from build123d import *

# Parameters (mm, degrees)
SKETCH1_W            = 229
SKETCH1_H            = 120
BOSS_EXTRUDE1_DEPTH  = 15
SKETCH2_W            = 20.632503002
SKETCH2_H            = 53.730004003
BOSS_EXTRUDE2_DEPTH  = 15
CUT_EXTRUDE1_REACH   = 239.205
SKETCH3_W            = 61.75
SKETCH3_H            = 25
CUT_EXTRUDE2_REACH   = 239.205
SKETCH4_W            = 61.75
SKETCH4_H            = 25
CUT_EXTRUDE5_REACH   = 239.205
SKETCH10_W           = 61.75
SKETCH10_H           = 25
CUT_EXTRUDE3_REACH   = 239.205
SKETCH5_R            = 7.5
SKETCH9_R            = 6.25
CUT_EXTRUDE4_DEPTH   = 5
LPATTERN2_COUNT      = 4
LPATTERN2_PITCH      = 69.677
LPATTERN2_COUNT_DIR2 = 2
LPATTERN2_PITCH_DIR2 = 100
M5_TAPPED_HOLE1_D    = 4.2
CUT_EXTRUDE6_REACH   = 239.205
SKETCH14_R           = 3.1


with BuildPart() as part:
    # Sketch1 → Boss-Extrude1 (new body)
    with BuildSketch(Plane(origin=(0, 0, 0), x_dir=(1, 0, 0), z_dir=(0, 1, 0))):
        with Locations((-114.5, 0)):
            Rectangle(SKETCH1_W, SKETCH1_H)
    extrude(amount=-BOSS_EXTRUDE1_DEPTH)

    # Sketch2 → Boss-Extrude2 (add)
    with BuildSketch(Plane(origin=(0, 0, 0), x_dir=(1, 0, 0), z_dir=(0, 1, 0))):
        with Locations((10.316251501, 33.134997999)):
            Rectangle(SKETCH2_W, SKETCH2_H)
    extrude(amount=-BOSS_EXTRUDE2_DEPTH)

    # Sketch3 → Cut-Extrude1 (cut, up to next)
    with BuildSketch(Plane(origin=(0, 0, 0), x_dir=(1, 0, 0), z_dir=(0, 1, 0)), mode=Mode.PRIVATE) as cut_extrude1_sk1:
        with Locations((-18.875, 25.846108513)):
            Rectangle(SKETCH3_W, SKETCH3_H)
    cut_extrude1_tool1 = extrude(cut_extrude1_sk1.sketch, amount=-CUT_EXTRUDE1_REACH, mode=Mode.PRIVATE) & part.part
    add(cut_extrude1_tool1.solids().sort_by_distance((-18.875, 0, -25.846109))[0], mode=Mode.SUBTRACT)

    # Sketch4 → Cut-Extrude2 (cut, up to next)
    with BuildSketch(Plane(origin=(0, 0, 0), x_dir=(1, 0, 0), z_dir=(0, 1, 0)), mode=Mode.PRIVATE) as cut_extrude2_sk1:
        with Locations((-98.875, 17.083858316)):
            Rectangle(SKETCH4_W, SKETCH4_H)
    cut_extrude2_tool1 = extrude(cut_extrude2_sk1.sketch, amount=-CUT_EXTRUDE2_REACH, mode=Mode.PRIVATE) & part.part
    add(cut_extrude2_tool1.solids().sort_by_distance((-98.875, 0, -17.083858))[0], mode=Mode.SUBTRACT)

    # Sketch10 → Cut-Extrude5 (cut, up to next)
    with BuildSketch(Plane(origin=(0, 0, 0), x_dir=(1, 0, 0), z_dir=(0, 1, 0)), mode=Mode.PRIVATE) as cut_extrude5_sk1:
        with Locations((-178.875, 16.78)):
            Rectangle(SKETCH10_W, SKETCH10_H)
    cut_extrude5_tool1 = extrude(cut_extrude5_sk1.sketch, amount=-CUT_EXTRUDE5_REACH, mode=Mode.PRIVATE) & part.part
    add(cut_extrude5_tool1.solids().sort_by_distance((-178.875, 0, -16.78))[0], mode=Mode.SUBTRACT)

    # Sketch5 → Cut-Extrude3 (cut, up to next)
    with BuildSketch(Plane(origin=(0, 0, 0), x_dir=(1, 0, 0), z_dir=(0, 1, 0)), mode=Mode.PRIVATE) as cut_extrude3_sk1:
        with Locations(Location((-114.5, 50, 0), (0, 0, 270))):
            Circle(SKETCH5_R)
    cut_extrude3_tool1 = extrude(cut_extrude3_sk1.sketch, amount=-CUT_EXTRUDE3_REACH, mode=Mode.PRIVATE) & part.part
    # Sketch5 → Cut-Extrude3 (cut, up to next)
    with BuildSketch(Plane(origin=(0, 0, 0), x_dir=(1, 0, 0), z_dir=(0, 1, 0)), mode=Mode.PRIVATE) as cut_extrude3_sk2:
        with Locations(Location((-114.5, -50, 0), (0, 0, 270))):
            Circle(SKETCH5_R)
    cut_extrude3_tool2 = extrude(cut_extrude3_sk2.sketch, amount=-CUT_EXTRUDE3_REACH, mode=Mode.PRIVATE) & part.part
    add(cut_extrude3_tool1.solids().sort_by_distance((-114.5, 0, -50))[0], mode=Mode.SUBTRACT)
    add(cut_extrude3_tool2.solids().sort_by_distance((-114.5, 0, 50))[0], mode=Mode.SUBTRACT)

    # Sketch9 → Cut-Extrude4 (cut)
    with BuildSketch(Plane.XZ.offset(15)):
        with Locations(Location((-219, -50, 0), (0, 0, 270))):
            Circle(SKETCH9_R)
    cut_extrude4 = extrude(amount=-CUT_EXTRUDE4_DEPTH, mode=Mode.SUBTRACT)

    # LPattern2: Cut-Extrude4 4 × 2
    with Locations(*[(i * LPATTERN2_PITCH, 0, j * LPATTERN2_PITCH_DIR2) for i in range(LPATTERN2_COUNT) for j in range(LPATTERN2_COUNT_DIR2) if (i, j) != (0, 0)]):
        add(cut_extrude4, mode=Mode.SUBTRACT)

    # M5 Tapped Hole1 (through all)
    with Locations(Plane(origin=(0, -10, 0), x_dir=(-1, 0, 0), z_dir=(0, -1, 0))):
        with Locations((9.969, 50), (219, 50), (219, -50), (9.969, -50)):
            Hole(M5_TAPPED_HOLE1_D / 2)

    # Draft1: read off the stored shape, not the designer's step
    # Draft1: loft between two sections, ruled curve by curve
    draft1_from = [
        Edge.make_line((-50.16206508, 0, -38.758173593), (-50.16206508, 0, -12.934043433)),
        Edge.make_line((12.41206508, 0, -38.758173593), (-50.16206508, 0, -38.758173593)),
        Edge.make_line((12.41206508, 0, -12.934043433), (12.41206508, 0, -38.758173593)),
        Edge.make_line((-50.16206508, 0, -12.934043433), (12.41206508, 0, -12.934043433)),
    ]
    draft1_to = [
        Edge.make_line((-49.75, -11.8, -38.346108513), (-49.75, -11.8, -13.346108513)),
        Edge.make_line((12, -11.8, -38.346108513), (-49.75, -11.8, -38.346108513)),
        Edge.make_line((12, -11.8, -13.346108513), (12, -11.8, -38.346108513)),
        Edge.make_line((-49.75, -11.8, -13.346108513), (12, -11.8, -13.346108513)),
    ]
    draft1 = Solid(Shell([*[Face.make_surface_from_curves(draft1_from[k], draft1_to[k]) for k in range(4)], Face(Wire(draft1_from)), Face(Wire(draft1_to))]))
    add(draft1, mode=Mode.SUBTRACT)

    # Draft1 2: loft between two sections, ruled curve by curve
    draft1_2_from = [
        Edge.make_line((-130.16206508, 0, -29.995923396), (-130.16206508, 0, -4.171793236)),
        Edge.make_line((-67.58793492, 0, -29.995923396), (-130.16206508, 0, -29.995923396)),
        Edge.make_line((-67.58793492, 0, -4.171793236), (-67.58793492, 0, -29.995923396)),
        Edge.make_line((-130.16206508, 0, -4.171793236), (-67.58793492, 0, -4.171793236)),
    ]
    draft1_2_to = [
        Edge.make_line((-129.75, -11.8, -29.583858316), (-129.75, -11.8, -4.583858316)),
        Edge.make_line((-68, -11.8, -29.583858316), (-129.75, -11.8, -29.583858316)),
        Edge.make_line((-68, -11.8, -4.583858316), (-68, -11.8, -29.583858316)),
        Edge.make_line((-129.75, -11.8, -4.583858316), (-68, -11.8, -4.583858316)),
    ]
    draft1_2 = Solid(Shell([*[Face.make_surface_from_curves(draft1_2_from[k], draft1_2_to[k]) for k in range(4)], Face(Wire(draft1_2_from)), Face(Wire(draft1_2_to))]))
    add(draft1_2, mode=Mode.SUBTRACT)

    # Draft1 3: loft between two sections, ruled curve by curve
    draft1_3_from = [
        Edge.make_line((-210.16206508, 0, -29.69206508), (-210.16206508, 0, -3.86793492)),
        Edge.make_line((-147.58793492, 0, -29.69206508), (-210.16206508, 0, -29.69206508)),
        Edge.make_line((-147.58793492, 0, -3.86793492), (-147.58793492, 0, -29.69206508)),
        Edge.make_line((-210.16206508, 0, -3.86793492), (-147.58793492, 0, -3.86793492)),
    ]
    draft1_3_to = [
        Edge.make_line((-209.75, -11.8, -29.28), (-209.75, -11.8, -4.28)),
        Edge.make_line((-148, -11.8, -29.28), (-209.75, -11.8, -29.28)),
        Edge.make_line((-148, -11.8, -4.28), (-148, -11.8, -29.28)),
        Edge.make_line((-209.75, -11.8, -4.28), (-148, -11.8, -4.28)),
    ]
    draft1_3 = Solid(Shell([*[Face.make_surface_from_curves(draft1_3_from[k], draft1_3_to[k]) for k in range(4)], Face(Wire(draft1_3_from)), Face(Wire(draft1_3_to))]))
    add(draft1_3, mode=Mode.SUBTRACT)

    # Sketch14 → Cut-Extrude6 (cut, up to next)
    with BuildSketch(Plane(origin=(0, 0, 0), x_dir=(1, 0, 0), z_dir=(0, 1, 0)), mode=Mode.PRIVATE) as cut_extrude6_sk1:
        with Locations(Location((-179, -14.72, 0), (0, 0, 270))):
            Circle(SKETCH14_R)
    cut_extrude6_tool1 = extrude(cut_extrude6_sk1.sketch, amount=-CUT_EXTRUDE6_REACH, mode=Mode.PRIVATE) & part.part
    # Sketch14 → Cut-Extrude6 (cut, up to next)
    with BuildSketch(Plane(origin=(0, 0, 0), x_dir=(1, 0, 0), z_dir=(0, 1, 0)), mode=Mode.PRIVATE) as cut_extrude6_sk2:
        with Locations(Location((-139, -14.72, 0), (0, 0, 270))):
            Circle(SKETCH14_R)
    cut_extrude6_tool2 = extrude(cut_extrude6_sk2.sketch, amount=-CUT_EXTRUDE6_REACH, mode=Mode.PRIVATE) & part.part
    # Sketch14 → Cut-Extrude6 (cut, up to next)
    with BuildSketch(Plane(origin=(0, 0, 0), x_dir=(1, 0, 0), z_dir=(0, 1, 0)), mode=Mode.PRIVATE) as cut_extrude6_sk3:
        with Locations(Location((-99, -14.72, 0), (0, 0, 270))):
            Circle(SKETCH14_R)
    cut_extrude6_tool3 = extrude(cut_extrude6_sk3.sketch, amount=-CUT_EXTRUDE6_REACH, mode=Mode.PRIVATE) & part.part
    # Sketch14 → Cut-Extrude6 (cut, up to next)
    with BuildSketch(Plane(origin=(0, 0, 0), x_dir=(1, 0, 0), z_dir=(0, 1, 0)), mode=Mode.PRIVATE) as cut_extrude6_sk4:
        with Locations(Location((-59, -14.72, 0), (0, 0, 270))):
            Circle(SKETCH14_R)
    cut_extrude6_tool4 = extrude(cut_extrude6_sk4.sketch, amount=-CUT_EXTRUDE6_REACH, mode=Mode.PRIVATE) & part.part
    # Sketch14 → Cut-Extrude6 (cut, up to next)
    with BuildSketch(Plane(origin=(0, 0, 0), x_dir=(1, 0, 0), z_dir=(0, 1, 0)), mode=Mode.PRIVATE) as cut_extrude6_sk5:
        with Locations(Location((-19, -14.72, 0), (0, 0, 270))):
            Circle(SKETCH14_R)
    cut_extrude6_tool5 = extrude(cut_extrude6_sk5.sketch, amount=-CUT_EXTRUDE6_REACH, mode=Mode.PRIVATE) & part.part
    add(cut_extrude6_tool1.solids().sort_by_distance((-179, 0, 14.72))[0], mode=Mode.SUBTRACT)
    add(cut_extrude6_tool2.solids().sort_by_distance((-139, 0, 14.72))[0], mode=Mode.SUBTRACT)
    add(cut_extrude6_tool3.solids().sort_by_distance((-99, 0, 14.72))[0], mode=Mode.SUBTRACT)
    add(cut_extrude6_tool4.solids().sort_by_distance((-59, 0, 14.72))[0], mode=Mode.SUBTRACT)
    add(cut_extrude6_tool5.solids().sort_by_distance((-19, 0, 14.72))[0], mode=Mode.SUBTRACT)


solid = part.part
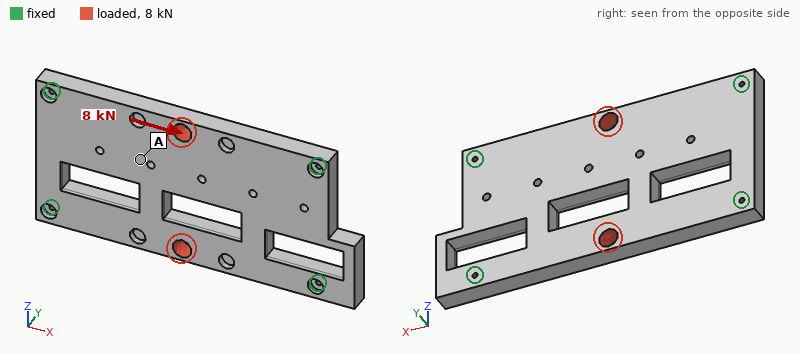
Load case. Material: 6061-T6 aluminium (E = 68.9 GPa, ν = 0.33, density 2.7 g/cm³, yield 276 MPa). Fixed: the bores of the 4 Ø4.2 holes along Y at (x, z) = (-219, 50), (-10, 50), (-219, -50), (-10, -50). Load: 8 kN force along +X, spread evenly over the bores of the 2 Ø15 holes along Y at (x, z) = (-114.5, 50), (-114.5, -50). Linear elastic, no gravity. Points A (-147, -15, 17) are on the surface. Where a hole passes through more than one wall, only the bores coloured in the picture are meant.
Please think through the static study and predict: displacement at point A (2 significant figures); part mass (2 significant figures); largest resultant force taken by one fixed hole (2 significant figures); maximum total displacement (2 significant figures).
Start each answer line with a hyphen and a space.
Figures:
- 5.3 µm
- 930 g
- 2.1 kN
- 10 µm
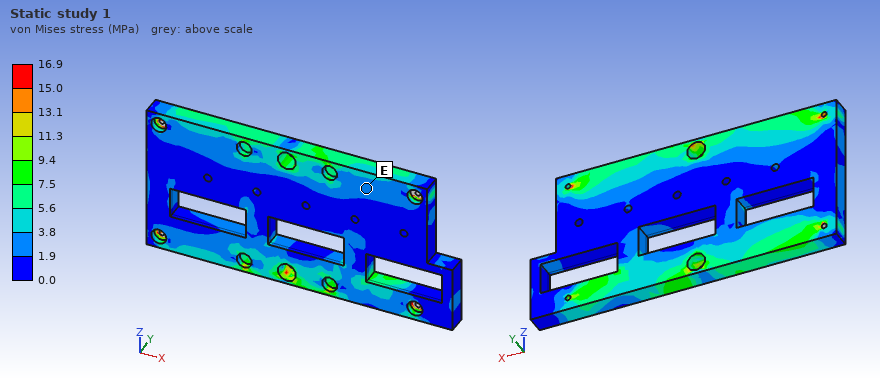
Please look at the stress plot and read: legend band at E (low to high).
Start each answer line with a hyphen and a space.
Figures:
- 1.9 to 3.8 MPa
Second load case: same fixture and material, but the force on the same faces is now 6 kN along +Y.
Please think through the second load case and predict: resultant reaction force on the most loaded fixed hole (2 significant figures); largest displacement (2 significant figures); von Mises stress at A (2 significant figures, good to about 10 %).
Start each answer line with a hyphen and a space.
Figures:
- 2.4 kN
- 0.43 mm
- 24 MPa
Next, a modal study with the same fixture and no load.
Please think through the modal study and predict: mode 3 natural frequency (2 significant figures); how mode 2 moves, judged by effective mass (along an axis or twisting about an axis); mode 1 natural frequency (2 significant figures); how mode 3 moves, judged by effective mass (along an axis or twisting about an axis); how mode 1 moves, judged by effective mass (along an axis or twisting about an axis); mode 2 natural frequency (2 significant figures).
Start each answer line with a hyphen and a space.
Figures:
- 3000 Hz
- twisting about X
- 1100 Hz
- twisting about Z
- along Y
- 2000 Hz
